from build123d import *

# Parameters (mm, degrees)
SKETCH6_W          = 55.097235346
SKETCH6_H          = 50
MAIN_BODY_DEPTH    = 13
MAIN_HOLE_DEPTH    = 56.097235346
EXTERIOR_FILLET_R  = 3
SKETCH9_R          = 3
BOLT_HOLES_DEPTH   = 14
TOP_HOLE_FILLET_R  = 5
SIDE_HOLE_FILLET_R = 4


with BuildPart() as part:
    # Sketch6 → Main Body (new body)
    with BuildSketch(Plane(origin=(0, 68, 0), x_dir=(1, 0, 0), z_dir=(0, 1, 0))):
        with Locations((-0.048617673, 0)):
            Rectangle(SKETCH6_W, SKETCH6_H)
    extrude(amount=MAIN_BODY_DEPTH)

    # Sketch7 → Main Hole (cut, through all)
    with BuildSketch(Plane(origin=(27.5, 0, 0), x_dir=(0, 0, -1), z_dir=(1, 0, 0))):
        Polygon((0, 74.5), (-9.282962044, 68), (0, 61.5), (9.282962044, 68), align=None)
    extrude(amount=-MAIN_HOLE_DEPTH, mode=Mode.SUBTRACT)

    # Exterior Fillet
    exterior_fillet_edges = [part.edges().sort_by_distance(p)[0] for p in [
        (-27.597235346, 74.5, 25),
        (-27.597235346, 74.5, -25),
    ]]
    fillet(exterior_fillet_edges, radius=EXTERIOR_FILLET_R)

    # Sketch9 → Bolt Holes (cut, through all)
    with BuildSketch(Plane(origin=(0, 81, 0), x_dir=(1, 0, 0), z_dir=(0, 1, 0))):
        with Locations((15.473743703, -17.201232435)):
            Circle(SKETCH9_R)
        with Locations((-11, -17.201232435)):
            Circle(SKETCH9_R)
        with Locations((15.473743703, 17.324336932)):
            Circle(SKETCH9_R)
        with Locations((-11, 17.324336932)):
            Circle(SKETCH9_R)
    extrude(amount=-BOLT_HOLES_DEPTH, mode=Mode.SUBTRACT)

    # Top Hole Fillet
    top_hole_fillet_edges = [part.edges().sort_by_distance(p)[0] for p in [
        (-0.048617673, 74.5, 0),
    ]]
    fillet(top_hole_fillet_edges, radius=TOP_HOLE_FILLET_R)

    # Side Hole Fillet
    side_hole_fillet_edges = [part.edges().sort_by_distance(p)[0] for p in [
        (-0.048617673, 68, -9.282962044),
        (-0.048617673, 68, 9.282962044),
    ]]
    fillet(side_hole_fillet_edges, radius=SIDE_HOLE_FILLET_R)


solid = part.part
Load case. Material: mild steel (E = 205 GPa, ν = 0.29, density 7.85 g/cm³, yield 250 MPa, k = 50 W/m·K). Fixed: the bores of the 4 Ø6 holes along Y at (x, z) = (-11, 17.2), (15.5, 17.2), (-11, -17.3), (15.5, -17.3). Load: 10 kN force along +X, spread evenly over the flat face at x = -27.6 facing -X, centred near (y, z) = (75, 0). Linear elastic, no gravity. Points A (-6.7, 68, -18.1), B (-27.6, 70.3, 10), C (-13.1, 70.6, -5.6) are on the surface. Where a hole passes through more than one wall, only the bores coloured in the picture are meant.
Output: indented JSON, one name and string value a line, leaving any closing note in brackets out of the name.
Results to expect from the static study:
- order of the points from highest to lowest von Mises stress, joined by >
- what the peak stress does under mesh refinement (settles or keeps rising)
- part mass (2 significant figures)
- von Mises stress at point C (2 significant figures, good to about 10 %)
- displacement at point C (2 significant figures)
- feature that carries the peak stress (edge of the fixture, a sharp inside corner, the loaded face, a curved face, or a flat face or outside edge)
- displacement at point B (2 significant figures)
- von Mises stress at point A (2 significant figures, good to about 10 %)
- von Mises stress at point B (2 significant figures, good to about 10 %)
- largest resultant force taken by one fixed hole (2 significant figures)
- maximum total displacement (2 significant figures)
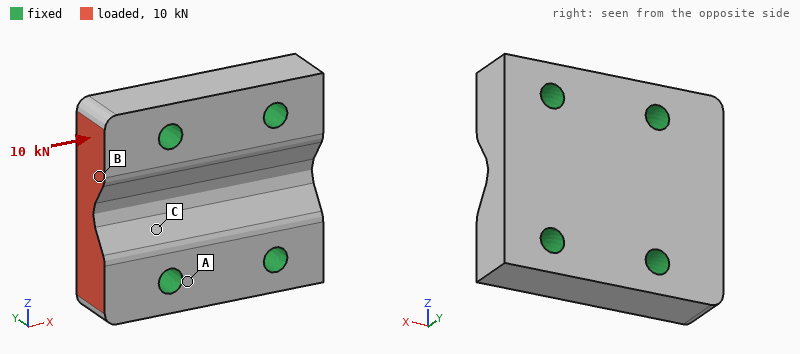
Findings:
{
  "order of the points from highest to lowest von Mises stress, joined by >": "B > C > A",
  "what the peak stress does under mesh refinement": "keeps rising",
  "part mass": "240 g",
  "von Mises stress at point C": "11 MPa",
  "displacement at point C": "0.99 µm",
  "feature that carries the peak stress": "edge of the fixture",
  "displacement at point B": "2.0 µm",
  "von Mises stress at point A": "5.2 MPa",
  "von Mises stress at point B": "18 MPa",
  "largest resultant force taken by one fixed hole": "4.3 kN",
  "maximum total displacement": "2.6 µm"
}
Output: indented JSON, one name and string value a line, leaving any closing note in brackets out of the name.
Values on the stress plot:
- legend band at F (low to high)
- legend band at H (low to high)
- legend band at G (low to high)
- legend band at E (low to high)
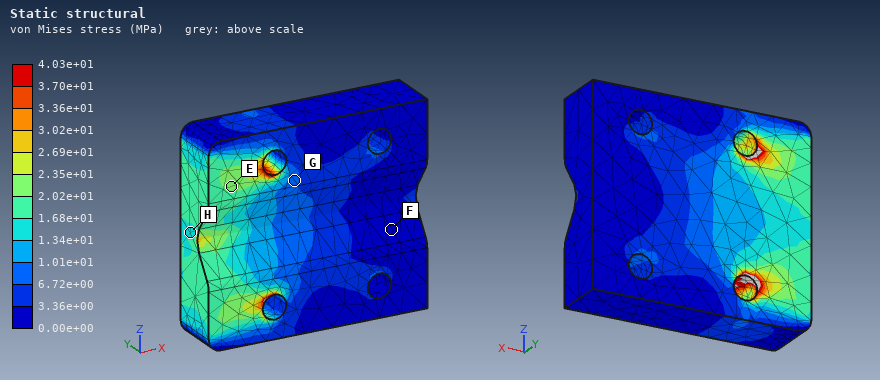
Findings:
{
  "legend band at F": "0.00e+00 to 3.36e+00 MPa",
  "legend band at H": "1.34e+01 to 1.68e+01 MPa",
  "legend band at G": "6.72e+00 to 1.01e+01 MPa",
  "legend band at E": "2.02e+01 to 2.35e+01 MPa"
}
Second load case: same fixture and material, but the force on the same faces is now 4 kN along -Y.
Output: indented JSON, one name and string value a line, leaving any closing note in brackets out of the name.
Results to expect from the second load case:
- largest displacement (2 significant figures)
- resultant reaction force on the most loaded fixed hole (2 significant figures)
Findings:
{
  "largest displacement": "8.2 µm",
  "resultant reaction force on the most loaded fixed hole": "2.3 kN"
}
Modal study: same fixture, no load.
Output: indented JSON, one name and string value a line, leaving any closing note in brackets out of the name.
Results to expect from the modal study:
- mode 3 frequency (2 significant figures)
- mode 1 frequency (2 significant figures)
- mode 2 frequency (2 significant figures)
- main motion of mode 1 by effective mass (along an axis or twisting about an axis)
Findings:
{
  "mode 3 frequency": "34 kHz",
  "mode 1 frequency": "26 kHz",
  "mode 2 frequency": "33 kHz",
  "main motion of mode 1 by effective mass": "along Y"
}
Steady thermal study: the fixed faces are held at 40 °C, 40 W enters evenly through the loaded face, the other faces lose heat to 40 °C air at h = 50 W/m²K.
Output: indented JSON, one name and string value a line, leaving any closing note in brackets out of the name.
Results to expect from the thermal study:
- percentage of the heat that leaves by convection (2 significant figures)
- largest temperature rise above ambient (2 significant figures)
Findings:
{
  "percentage of the heat that leaves by convection": "3.8 %",
  "largest temperature rise above ambient": "26 K"
}
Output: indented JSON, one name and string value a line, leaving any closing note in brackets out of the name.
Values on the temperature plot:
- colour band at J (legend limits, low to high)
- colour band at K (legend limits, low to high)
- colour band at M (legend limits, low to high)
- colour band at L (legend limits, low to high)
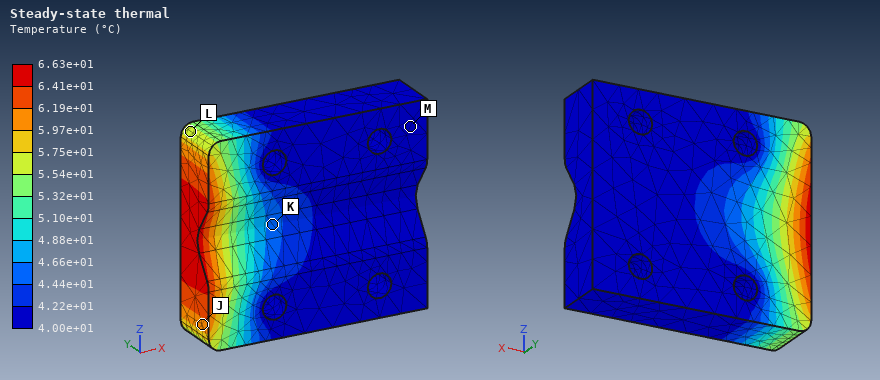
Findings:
{
  "colour band at J": "5.97e+01 to 6.19e+01 °C",
  "colour band at K": "4.44e+01 to 4.66e+01 °C",
  "colour band at M": "4.00e+01 to 4.22e+01 °C",
  "colour band at L": "5.54e+01 to 5.75e+01 °C"
}
